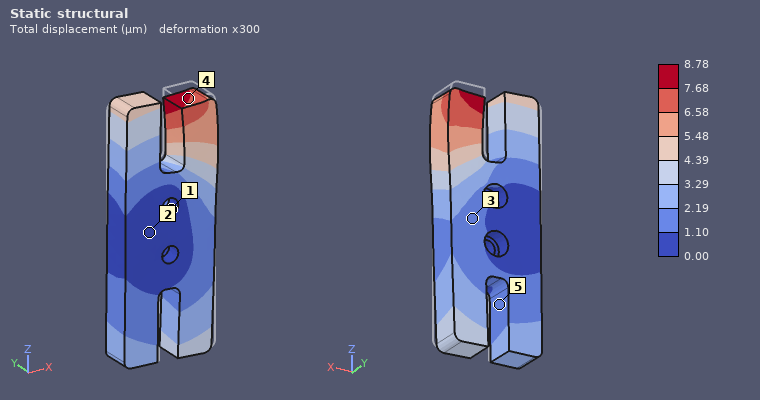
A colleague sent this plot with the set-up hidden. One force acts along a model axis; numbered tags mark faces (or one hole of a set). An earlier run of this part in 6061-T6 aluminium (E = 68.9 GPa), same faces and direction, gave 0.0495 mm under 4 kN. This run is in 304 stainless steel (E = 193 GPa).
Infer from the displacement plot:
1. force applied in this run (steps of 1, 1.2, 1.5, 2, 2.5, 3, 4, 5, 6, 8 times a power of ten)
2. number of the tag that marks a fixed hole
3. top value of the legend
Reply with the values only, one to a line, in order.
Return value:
2 kN
1
8.78 µm
